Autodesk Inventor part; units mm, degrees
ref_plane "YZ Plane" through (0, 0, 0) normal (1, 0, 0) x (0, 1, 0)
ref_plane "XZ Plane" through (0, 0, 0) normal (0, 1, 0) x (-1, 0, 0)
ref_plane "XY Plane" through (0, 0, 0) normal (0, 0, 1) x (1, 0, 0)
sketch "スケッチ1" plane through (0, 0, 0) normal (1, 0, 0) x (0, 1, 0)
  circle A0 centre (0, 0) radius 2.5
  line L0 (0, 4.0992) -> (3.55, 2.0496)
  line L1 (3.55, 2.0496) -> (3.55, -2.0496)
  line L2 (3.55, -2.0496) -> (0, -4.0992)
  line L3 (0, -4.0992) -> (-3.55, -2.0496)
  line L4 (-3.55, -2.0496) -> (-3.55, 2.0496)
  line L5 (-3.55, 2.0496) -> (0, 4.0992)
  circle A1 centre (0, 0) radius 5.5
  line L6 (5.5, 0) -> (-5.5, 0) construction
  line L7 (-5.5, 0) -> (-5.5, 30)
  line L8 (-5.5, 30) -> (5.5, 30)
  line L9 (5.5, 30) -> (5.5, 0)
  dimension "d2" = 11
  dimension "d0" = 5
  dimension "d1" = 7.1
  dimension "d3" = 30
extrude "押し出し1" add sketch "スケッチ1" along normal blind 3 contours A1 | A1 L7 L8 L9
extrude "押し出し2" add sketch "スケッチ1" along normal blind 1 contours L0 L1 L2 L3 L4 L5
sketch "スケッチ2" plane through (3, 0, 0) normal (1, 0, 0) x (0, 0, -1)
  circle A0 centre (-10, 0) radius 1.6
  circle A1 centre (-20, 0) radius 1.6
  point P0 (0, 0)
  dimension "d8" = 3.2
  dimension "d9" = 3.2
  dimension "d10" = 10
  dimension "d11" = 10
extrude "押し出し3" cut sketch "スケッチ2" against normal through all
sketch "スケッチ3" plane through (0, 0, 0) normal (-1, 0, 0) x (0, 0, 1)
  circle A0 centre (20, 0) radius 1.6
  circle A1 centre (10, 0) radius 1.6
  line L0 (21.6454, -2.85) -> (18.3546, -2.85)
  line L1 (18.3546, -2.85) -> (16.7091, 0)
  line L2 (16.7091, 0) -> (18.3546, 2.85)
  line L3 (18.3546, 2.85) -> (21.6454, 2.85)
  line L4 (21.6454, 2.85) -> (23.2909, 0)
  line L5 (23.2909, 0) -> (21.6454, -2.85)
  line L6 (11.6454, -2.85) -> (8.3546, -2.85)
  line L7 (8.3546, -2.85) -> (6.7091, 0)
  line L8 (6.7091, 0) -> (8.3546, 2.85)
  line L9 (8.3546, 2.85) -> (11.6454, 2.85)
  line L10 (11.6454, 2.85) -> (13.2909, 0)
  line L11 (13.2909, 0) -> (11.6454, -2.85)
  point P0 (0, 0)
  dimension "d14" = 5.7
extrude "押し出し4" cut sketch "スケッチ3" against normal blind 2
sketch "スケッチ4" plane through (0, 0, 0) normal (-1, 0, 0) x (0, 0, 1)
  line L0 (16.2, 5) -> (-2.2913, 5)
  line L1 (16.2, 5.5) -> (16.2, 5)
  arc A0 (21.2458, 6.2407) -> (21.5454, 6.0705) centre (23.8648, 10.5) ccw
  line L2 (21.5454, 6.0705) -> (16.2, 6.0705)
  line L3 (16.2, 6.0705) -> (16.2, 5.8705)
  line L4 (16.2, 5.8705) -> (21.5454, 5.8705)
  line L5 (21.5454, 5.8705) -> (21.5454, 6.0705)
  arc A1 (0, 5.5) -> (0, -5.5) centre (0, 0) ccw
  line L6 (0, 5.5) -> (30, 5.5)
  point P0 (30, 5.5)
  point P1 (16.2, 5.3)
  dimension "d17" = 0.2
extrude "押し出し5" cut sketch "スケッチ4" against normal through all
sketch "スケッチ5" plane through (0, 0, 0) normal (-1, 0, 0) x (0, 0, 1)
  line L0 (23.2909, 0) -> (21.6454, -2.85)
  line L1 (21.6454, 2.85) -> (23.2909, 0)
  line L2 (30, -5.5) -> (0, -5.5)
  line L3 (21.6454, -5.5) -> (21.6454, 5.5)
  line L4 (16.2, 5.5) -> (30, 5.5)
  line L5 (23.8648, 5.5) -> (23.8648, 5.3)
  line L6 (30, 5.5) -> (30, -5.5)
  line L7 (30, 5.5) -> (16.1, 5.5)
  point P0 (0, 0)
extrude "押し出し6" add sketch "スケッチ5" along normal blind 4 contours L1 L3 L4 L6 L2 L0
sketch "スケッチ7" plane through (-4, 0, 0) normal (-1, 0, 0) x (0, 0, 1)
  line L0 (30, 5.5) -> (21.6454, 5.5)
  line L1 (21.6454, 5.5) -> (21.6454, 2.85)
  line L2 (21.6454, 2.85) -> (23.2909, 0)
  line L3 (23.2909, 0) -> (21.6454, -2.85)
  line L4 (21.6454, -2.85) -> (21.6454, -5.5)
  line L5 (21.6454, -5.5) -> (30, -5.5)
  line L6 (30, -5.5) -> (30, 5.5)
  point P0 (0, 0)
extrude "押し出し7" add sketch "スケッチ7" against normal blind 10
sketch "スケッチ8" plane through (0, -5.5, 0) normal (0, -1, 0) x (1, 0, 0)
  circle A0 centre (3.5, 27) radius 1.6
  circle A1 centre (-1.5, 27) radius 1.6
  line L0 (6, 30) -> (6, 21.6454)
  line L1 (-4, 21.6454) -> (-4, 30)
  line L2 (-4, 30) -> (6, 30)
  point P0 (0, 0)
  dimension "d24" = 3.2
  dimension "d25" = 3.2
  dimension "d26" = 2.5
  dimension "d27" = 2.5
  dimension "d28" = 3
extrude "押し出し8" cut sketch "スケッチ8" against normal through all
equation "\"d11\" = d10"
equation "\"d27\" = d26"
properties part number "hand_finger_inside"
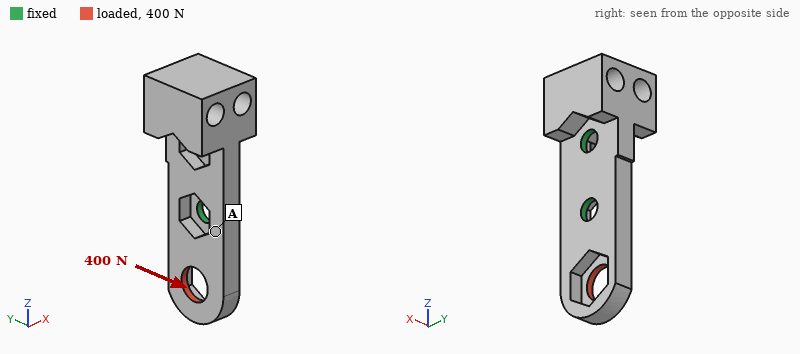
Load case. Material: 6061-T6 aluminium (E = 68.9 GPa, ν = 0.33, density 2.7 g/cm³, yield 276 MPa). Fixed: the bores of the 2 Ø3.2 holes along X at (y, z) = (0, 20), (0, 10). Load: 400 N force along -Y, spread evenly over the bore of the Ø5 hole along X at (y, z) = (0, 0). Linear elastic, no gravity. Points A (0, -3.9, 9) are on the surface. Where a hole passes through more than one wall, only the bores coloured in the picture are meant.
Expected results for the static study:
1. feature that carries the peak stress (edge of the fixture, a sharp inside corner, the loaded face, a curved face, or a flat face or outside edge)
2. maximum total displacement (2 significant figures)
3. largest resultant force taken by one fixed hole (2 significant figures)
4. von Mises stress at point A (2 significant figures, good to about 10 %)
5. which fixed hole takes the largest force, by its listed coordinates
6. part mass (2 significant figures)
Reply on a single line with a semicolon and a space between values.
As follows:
edge of the fixture; 63 µm; 630 N; 36 MPa; (0, 10); 3.5 g
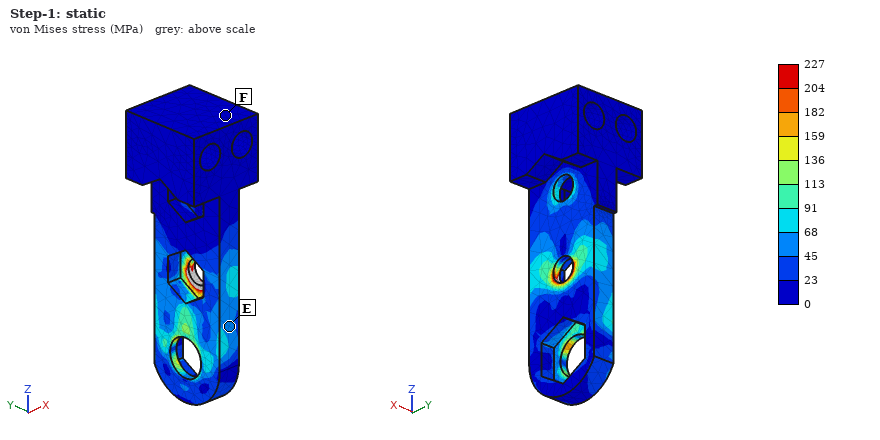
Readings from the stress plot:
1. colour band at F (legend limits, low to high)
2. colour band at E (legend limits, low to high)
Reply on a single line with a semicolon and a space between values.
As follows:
0 to 23 MPa; 45 to 68 MPa
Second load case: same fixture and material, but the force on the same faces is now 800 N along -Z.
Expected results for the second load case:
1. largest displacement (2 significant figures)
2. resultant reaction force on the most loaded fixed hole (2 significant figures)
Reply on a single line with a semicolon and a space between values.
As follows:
0.12 mm; 430 N
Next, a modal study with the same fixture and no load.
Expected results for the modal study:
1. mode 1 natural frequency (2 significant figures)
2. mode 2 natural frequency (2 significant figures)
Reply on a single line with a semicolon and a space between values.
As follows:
9600 Hz; 9800 Hz
